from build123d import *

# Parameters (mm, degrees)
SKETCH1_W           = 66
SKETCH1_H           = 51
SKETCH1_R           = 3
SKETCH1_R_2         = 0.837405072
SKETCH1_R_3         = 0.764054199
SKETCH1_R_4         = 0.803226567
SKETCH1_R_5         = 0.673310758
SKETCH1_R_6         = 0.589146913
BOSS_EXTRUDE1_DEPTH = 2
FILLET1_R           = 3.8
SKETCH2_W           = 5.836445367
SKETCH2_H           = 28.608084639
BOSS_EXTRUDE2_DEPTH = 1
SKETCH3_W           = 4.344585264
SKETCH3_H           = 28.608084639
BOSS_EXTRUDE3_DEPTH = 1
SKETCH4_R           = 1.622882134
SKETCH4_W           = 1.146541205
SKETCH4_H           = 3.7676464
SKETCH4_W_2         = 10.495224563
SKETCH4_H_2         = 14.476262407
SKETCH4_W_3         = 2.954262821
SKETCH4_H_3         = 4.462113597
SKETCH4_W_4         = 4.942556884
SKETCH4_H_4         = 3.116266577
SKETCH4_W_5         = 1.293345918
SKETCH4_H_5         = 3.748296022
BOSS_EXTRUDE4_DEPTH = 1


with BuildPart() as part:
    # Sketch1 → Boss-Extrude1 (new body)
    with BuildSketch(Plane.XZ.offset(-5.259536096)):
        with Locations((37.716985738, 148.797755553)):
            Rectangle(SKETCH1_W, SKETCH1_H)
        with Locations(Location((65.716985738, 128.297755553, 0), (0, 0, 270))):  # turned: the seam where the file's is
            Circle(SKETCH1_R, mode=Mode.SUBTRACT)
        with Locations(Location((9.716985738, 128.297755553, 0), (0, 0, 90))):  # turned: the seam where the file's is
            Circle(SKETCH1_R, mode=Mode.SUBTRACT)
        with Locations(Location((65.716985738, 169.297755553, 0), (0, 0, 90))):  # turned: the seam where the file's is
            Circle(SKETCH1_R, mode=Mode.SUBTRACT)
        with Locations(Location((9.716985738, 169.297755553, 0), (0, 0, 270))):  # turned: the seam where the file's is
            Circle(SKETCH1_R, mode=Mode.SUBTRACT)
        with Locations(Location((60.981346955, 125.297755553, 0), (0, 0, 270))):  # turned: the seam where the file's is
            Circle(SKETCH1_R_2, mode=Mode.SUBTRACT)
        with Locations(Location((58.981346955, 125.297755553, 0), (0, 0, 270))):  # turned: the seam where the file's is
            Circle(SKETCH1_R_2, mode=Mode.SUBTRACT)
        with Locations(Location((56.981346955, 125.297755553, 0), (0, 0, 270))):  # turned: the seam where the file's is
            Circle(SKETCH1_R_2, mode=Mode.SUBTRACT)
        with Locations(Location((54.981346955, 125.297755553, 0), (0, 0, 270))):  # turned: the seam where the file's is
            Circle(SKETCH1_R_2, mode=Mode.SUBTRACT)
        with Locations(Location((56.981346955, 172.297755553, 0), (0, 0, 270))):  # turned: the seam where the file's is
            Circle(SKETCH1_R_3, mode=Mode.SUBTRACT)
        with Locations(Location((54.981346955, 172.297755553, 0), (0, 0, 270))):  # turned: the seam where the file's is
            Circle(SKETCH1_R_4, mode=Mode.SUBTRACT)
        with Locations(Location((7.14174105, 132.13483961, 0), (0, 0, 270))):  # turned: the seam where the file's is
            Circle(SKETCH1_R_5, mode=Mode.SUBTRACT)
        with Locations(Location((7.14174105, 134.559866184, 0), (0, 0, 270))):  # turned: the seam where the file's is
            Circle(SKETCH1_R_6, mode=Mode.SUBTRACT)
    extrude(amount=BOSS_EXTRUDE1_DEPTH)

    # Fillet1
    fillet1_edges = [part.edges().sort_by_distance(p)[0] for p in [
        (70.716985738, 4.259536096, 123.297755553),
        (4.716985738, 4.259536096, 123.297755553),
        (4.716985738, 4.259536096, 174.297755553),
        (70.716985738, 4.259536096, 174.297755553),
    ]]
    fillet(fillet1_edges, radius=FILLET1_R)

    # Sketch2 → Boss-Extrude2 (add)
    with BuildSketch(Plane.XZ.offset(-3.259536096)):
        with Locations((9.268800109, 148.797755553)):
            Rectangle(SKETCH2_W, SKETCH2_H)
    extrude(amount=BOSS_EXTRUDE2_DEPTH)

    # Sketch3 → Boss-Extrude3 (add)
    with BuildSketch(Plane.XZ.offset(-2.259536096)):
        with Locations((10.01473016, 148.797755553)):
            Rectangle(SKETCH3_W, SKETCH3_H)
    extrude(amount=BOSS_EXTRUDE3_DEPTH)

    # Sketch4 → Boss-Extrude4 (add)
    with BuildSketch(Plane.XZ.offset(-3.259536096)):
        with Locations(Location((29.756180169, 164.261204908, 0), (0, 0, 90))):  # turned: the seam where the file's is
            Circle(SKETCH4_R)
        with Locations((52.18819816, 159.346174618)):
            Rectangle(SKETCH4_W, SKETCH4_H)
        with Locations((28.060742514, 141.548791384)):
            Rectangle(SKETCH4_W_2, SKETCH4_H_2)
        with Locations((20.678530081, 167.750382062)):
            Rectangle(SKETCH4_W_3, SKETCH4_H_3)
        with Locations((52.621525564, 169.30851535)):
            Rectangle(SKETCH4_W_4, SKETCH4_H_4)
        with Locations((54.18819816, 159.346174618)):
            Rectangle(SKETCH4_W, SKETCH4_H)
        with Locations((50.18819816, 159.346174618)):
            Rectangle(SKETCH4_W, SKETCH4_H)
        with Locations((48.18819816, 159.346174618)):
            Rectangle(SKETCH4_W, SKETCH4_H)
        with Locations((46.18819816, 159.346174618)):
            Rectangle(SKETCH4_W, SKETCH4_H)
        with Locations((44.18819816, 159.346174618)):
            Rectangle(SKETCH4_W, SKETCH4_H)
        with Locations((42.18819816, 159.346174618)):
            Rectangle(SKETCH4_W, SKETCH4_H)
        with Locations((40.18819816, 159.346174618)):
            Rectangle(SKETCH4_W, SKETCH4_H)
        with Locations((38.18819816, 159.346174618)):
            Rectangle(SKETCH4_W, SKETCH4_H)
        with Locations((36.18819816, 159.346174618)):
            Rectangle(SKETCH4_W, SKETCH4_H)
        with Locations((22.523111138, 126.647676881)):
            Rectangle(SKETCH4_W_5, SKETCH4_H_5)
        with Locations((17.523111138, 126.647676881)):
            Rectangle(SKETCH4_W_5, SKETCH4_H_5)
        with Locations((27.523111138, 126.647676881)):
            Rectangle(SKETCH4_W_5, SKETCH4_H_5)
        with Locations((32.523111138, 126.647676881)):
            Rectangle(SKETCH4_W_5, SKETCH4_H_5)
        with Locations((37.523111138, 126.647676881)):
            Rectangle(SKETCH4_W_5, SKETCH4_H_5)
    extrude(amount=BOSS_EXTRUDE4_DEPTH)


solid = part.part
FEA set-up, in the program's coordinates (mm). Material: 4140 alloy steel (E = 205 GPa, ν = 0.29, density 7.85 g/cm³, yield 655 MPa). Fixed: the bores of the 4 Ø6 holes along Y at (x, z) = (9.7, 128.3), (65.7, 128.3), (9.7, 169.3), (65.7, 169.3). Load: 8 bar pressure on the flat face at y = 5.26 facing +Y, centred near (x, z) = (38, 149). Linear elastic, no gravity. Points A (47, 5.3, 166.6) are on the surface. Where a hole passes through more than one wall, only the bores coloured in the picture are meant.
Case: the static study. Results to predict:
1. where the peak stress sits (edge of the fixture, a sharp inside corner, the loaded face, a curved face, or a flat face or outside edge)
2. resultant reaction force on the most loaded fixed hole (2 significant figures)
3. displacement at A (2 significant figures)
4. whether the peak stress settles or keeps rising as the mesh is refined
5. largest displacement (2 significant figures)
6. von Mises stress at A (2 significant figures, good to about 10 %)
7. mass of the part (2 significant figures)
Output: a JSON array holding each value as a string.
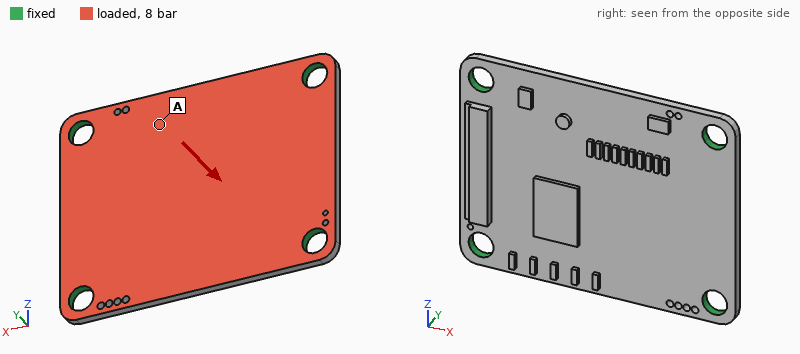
["a sharp inside corner", "730 N", "0.11 mm", "keeps rising", "0.17 mm", "110 MPa", "55 g"]
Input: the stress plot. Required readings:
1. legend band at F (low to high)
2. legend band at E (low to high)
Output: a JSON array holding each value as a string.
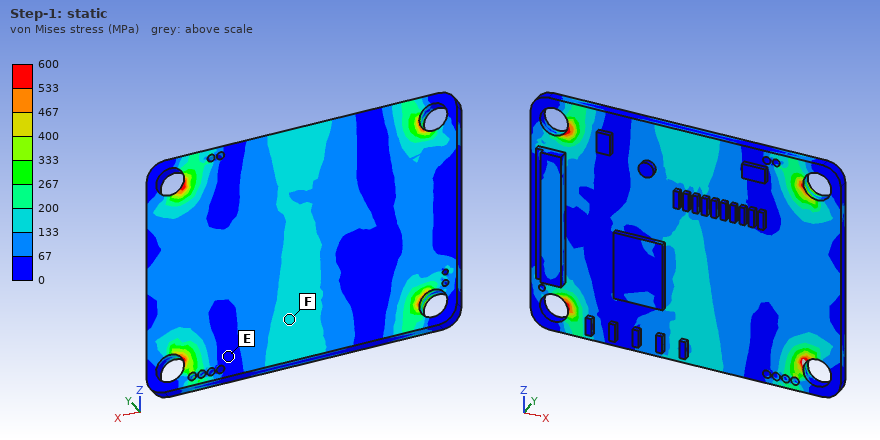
["133 to 200 MPa", "0 to 67 MPa"]
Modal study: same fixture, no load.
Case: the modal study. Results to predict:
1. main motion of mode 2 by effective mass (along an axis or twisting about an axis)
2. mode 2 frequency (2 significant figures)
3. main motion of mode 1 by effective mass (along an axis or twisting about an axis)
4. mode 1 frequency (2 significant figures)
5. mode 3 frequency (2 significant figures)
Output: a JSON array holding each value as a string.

["twisting about X", "4700 Hz", "along Y", "3200 Hz", "6900 Hz"]
